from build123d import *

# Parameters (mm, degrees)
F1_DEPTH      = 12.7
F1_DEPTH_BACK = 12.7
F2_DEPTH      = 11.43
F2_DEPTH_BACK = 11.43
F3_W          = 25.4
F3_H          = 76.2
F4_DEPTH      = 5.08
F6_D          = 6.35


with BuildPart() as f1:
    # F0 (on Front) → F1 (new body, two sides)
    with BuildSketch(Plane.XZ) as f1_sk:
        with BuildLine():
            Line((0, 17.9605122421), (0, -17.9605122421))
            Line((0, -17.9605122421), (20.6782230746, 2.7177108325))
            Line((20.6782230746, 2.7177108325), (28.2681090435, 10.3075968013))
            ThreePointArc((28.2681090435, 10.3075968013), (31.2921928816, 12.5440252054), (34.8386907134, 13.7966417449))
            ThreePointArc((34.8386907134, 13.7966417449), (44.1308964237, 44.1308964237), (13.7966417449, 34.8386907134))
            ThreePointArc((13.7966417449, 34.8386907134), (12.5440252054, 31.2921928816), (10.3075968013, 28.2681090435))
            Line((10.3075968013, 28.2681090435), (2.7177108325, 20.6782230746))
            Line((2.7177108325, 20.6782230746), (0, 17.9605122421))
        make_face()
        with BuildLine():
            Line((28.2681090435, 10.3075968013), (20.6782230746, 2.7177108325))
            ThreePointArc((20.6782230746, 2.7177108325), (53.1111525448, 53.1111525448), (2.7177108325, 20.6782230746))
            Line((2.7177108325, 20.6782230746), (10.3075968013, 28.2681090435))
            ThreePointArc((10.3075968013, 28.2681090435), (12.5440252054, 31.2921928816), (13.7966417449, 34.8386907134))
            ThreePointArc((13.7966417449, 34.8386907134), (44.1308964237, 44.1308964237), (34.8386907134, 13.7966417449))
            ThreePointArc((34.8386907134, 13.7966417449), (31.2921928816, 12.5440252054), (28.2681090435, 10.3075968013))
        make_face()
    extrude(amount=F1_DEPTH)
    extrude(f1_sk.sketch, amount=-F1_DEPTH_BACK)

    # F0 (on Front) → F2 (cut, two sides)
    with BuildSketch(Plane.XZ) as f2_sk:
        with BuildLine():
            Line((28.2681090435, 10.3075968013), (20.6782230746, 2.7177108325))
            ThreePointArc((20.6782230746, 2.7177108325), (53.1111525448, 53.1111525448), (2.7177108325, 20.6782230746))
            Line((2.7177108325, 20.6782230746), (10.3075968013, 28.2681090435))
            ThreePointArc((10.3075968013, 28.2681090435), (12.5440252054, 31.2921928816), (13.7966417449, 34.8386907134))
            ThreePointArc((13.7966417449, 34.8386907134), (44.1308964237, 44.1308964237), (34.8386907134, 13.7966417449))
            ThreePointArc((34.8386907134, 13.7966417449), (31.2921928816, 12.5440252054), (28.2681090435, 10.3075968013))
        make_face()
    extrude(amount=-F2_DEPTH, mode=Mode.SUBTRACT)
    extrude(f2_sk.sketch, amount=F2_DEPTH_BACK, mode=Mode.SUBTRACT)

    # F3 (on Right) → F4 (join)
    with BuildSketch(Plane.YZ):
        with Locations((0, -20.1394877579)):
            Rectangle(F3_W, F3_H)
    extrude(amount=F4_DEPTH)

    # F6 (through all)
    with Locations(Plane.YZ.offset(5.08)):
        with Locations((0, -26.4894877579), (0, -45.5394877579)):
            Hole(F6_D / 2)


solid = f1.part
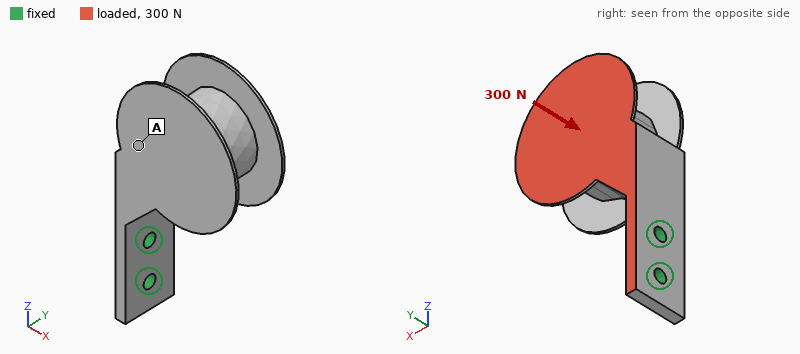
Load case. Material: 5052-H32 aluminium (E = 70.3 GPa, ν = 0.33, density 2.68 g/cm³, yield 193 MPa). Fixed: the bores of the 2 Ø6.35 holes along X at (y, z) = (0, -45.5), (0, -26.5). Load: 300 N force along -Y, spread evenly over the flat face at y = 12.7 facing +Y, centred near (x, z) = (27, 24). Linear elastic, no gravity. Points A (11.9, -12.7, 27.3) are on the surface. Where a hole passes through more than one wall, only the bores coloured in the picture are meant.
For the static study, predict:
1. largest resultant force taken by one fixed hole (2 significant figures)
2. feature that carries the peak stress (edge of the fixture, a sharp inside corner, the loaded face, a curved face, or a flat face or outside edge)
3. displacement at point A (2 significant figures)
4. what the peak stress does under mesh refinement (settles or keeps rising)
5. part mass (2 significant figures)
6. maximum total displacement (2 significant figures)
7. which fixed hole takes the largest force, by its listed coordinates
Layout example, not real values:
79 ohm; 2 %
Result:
750 N; edge of the fixture; 0.076 mm; keeps rising; 140 g; 0.24 mm; (0, -26.5)
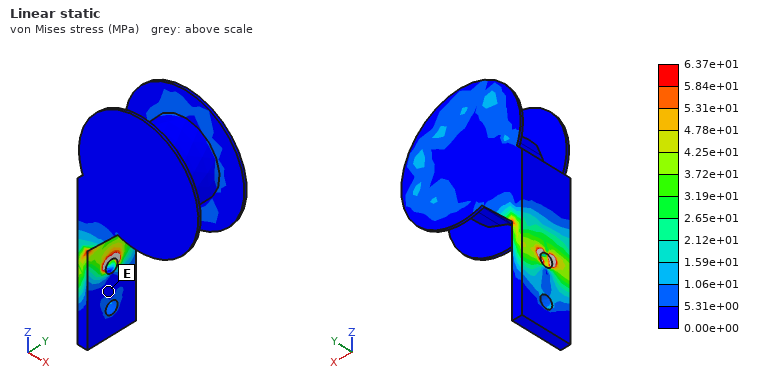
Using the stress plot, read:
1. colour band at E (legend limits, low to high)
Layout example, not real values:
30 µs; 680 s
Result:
0.00e+00 to 5.31e+00 MPa
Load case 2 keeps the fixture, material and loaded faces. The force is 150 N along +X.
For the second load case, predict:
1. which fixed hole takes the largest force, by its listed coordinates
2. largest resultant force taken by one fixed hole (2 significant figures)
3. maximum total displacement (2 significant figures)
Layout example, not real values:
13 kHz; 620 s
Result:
(0, -26.5); 230 N; 0.46 mm
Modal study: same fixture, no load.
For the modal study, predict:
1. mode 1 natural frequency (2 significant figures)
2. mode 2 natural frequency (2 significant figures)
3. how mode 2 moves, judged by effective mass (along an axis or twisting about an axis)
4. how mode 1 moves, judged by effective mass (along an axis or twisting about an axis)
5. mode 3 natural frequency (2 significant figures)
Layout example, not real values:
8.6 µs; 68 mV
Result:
310 Hz; 710 Hz; along Y; along X; 2300 Hz
